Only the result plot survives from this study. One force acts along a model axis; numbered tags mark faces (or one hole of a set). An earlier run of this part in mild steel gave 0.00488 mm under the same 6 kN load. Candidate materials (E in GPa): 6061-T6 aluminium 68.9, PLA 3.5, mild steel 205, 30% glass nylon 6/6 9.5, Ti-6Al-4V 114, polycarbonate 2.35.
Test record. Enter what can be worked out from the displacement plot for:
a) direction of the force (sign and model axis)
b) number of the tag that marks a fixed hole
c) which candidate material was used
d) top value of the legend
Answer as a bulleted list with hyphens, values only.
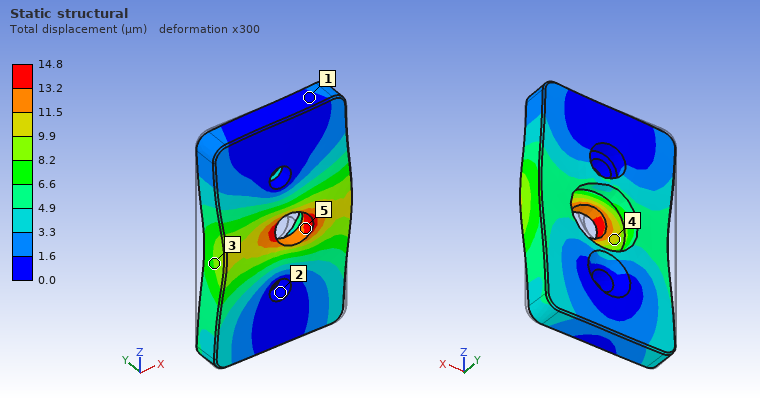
- +X
- 2
- 6061-T6 aluminium
- 14.8 µm
